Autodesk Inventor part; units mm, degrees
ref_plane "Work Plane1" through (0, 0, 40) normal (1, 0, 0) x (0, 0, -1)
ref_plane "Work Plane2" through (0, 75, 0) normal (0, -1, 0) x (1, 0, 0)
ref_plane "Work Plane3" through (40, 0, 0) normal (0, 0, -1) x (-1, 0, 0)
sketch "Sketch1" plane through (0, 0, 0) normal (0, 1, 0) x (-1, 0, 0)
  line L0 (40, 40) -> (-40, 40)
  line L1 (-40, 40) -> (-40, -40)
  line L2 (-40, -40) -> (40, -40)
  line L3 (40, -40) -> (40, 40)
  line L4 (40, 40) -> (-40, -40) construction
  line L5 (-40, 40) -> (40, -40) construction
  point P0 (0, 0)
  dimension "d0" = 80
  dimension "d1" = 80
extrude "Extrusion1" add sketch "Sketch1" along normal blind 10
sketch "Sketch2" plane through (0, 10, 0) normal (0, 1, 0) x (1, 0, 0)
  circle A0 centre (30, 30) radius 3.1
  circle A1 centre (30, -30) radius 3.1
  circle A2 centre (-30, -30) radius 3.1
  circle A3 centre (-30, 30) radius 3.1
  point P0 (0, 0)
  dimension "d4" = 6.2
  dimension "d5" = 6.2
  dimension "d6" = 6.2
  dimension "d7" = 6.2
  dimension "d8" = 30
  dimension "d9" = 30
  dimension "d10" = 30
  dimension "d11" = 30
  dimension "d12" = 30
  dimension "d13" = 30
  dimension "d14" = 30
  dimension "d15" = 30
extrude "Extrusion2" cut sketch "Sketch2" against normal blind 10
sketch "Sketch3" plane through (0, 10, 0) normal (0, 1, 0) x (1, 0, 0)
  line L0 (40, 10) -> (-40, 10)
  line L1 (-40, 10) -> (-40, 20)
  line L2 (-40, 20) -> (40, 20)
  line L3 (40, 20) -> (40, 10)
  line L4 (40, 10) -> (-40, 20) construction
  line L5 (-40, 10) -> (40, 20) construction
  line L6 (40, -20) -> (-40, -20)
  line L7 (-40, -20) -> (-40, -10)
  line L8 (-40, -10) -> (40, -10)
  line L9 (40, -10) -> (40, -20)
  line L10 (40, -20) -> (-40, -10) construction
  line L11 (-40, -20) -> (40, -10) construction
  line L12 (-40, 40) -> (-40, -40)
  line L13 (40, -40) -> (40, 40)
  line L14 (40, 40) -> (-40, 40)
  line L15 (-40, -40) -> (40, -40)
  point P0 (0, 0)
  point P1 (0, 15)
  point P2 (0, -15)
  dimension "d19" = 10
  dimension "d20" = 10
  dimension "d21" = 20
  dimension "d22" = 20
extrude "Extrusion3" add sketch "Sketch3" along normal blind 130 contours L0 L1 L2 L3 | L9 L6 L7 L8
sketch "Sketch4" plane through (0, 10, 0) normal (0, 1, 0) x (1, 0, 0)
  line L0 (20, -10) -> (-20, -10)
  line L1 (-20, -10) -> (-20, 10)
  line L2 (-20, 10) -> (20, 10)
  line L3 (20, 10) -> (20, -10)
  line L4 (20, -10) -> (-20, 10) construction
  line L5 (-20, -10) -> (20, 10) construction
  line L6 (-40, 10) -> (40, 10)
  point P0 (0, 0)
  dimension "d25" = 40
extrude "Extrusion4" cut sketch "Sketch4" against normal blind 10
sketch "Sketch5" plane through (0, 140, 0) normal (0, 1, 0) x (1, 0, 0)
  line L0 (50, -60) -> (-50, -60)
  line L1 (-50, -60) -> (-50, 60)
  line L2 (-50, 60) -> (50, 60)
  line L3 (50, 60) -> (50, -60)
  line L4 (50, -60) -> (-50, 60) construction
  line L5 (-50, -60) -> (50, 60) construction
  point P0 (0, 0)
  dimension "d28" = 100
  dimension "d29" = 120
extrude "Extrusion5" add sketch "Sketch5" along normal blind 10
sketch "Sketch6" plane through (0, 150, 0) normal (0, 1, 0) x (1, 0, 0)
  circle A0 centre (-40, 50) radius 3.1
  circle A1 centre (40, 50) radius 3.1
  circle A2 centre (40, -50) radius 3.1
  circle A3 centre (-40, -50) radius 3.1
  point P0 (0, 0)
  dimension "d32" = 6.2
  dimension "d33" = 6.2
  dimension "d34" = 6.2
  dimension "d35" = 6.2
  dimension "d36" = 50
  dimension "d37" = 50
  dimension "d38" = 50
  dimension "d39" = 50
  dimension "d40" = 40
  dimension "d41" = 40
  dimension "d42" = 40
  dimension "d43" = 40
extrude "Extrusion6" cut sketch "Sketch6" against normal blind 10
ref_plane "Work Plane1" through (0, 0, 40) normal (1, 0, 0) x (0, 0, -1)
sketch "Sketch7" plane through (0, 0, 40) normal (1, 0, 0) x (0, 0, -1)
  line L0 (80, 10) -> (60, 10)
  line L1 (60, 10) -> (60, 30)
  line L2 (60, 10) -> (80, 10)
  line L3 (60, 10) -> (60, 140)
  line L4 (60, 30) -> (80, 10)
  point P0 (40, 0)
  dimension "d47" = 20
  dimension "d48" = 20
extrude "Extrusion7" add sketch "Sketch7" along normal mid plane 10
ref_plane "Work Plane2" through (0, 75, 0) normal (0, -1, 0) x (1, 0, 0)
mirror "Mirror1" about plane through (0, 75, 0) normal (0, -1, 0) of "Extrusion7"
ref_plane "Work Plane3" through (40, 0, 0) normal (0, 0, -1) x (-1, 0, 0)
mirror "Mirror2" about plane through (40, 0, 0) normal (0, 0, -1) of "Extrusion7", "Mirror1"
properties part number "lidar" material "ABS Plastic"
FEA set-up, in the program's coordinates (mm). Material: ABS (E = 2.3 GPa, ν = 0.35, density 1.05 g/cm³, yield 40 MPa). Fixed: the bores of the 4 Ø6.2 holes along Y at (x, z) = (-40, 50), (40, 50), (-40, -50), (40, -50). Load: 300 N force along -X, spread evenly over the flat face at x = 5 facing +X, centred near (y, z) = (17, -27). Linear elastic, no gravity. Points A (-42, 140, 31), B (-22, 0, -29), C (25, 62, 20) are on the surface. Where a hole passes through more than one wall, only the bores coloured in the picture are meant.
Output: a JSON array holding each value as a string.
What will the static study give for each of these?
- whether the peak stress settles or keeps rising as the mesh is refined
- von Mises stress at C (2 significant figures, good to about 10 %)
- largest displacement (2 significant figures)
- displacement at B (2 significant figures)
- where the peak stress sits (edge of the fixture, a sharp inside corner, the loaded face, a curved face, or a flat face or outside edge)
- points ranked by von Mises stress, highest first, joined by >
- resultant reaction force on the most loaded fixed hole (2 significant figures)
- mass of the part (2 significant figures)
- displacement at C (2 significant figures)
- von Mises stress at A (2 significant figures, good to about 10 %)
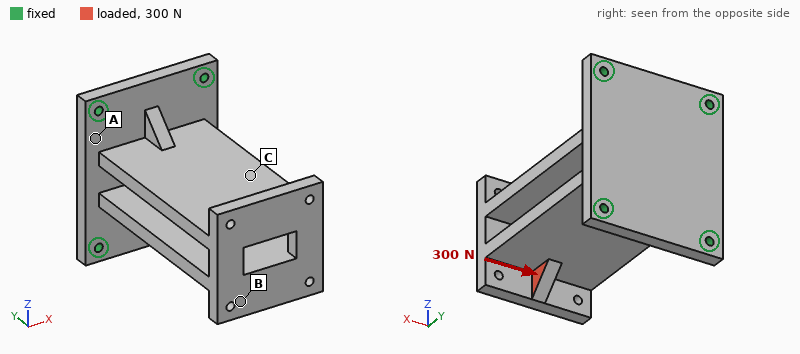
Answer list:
["keeps rising", "1.6 MPa", "1.4 mm", "1.3 mm", "edge of the fixture", "A > C > B", "300 N", "410 g", "0.47 mm", "2.6 MPa"]
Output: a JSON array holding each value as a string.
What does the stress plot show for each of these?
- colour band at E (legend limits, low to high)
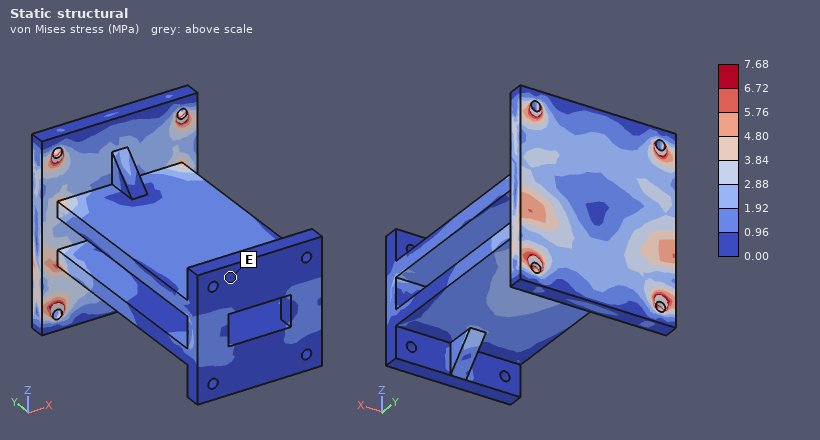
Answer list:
["0.00 to 0.96 MPa"]
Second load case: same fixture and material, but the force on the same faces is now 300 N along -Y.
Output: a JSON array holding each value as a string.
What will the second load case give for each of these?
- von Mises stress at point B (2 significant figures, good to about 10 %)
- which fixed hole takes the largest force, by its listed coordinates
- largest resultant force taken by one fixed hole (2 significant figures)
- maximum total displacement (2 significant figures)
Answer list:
["0.77 MPa", "(40, -50)", "130 N", "0.41 mm"]
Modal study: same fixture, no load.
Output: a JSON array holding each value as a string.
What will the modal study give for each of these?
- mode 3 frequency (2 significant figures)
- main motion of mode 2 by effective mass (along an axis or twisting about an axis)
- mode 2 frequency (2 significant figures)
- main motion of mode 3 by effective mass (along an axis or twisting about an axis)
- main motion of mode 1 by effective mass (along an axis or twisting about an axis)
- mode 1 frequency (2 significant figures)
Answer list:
["390 Hz", "along X", "230 Hz", "twisting about Y", "along Z", "150 Hz"]
